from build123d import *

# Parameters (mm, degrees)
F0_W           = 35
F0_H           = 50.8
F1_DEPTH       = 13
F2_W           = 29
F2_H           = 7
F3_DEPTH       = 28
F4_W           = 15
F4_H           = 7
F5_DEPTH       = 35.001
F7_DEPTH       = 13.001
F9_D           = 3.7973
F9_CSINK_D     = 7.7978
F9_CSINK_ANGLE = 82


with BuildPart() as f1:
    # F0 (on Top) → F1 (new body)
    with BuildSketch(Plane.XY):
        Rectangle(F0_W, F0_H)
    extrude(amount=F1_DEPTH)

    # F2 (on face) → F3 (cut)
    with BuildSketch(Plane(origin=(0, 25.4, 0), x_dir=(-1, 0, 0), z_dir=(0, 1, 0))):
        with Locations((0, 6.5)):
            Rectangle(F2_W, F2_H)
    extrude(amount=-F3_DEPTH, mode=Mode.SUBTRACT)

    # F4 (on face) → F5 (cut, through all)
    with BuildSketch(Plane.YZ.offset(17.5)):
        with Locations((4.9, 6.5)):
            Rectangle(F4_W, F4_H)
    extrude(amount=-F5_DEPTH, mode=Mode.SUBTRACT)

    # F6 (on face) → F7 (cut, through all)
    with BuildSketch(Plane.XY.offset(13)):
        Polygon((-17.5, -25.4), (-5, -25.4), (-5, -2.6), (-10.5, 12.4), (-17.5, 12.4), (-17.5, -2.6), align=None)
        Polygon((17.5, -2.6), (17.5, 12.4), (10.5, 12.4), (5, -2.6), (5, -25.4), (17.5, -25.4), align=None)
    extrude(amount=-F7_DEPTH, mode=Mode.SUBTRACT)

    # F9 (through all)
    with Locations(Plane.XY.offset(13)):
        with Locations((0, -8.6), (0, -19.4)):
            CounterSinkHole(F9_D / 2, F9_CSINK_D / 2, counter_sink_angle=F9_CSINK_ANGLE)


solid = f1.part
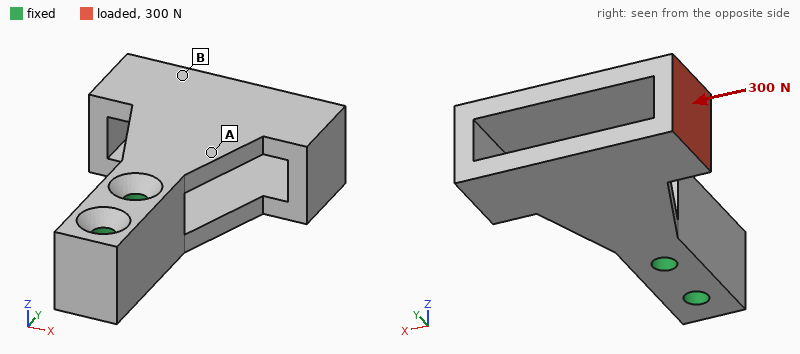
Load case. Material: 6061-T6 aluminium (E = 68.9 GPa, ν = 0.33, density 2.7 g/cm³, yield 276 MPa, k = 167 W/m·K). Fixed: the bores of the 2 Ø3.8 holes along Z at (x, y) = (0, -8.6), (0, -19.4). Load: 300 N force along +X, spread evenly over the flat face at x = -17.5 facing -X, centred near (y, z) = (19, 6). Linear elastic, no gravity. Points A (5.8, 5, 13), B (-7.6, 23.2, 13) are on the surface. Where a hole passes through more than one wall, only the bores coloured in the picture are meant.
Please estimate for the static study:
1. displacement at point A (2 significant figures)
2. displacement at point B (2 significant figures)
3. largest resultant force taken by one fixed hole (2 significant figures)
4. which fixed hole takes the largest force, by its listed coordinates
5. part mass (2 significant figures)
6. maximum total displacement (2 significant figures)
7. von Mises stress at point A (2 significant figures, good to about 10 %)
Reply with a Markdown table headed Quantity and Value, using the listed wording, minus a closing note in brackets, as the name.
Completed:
| Quantity | Value |
|---|---|
| displacement at point A | 22 µm |
| displacement at point B | 61 µm |
| largest resultant force taken by one fixed hole | 610 N |
| which fixed hole takes the largest force, by its listed coordinates | (0, -8.6) |
| part mass | 20 g |
| maximum total displacement | 75 µm |
| von Mises stress at point A | 14 MPa |
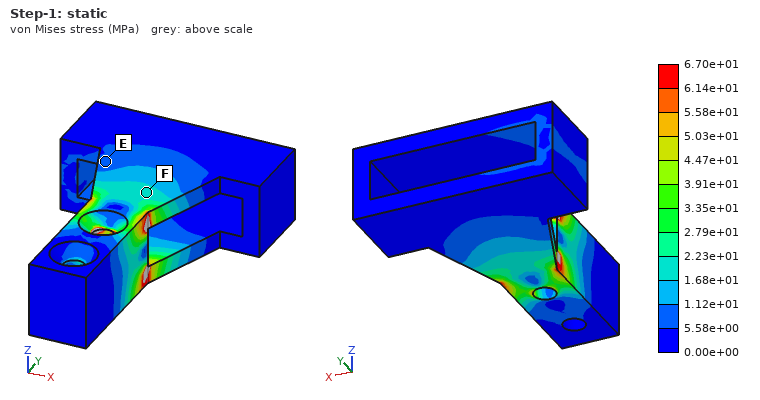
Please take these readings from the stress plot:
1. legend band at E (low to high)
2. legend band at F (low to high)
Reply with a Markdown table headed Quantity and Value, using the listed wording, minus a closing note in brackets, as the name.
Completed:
| Quantity | Value |
|---|---|
| legend band at E | 5.58e+00 to 1.12e+01 MPa |
| legend band at F | 1.68e+01 to 2.23e+01 MPa |
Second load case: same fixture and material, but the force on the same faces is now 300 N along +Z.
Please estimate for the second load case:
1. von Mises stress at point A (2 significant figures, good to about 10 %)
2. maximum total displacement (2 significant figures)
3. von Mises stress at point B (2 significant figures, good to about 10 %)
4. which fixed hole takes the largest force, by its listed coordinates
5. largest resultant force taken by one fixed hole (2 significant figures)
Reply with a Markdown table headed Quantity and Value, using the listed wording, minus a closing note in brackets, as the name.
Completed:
| Quantity | Value |
|---|---|
| von Mises stress at point A | 29 MPa |
| maximum total displacement | 0.21 mm |
| von Mises stress at point B | 29 MPa |
| which fixed hole takes the largest force, by its listed coordinates | (0, -8.6) |
| largest resultant force taken by one fixed hole | 410 N |
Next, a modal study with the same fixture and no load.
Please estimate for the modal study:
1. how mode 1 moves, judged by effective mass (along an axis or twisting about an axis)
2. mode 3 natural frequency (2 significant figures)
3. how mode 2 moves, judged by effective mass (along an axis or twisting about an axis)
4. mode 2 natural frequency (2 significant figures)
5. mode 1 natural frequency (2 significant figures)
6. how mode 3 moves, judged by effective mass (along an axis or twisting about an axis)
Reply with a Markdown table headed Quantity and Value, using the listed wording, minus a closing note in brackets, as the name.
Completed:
| Quantity | Value |
|---|---|
| how mode 1 moves, judged by effective mass | along Z |
| mode 3 natural frequency | 4300 Hz |
| how mode 2 moves, judged by effective mass | along X |
| mode 2 natural frequency | 3600 Hz |
| mode 1 natural frequency | 2700 Hz |
| how mode 3 moves, judged by effective mass | twisting about Y |
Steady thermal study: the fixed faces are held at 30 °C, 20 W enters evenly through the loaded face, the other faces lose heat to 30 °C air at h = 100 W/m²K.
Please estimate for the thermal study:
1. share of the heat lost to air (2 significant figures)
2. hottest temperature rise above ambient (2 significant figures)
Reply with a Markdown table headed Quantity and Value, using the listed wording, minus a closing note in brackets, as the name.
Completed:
| Quantity | Value |
|---|---|
| share of the heat lost to air | 35 % |
| hottest temperature rise above ambient | 40 K |
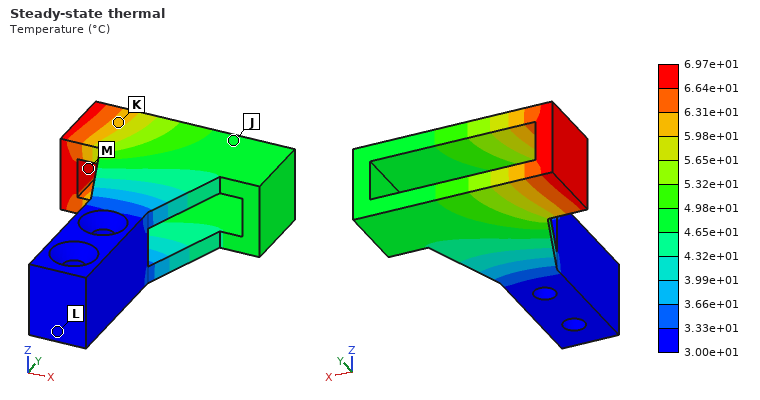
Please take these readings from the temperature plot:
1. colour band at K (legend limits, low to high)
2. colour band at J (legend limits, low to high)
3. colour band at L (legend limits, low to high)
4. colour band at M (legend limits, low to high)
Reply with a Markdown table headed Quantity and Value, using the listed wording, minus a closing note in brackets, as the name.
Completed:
| Quantity | Value |
|---|---|
| colour band at K | 5.98e+01 to 6.31e+01 °C |
| colour band at J | 4.65e+01 to 4.98e+01 °C |
| colour band at L | 3.00e+01 to 3.33e+01 °C |
| colour band at M | 6.64e+01 to 6.97e+01 °C |
